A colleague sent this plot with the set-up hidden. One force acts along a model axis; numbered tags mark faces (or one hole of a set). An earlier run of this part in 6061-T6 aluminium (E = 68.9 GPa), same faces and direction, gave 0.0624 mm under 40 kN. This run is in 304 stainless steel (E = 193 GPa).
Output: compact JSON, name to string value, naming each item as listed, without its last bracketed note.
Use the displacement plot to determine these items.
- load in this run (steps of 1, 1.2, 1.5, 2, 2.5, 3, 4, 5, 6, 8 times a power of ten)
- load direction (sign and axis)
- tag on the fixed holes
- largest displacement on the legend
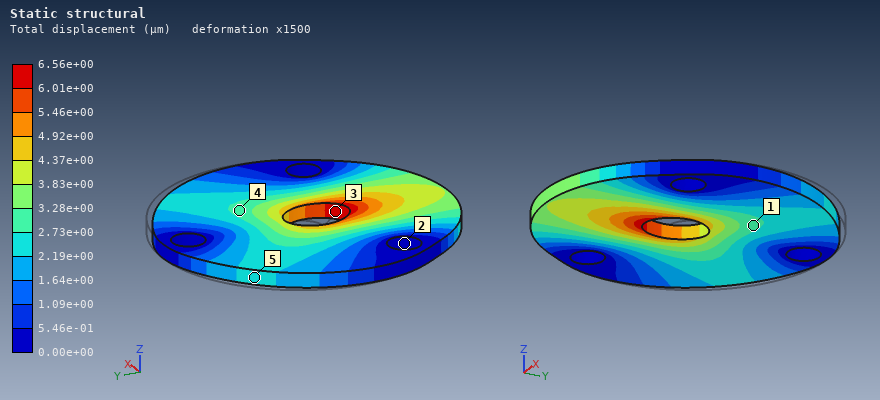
{"load in this run": "12 kN", "load direction": "-Y", "tag on the fixed holes": "2", "largest displacement on the legend": "6.56e+00 µm"}
